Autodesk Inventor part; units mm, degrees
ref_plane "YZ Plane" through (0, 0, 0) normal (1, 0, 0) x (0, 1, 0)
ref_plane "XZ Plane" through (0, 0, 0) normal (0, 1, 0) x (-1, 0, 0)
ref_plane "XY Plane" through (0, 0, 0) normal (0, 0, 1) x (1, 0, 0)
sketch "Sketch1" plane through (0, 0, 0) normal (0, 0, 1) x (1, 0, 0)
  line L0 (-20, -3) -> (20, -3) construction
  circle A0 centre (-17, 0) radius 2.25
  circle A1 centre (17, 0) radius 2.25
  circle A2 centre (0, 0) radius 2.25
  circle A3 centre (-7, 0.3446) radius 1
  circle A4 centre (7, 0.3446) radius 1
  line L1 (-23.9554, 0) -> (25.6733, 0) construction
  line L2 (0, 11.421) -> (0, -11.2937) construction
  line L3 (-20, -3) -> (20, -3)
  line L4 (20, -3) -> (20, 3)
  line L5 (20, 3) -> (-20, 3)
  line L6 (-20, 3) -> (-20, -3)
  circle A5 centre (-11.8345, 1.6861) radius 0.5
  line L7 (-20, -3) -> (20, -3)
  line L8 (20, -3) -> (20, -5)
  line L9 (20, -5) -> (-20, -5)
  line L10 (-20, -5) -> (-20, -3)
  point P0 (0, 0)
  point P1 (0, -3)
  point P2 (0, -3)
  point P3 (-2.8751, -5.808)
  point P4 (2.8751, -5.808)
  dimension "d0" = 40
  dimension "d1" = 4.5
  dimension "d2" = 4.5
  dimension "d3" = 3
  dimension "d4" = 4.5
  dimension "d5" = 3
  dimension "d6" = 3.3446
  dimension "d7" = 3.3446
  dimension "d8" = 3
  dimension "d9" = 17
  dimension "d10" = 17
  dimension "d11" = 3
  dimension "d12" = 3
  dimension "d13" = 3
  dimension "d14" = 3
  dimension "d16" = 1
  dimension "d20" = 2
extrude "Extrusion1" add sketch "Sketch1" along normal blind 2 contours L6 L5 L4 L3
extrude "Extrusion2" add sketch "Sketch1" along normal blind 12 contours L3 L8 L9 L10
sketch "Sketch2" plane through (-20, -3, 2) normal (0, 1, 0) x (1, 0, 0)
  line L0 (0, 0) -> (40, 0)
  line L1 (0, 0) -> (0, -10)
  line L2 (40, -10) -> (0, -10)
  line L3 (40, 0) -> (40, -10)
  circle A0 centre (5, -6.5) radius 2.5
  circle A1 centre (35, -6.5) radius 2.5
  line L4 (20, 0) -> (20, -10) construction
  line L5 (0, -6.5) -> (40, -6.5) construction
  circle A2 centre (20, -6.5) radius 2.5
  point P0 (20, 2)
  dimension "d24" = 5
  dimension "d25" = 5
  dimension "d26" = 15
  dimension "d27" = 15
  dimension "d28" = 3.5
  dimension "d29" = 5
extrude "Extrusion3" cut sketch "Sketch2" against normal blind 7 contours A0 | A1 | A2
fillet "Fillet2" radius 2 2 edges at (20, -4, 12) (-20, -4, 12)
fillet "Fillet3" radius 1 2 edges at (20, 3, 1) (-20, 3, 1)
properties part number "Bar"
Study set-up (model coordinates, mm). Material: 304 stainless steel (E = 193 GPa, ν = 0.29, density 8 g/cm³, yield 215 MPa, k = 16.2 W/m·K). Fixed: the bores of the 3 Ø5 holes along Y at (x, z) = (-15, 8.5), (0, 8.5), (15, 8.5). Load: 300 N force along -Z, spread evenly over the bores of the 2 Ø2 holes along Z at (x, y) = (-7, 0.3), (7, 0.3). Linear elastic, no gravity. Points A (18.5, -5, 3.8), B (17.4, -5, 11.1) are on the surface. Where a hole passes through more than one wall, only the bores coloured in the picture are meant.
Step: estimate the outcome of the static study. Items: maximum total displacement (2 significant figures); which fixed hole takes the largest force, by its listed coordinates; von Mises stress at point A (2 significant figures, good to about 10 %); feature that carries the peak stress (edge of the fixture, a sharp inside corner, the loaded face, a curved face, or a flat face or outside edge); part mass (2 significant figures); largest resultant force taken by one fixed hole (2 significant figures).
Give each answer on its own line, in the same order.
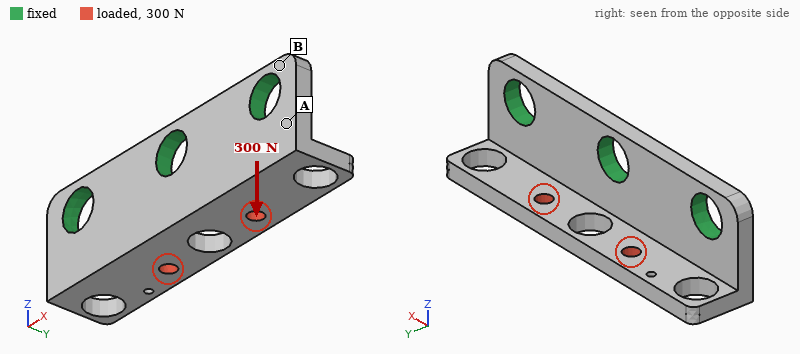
17 µm
(0, 8.5)
34 MPa
the loaded face
9.7 g
180 N
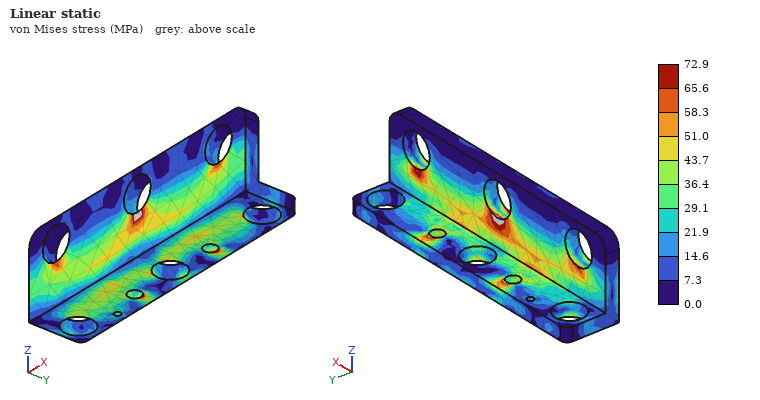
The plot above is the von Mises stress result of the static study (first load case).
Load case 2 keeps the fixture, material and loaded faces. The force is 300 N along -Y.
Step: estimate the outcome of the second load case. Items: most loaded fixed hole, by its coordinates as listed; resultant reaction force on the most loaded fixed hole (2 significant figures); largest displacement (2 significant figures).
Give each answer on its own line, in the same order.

(0, 8.5)
150 N
10 µm
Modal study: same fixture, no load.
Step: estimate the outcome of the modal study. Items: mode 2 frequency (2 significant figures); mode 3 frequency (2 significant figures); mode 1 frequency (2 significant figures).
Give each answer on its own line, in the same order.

17 kHz
29 kHz
14 kHz
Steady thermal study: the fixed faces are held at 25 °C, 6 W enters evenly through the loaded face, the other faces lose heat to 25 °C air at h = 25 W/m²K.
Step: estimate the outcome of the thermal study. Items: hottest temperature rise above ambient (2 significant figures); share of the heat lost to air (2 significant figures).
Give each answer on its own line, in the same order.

77 K
14 %
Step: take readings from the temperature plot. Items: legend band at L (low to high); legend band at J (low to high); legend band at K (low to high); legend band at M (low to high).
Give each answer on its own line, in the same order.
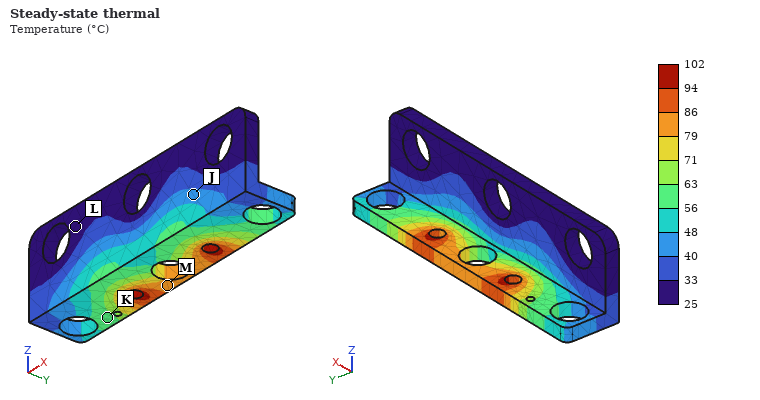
25 to 33 °C
40 to 48 °C
56 to 63 °C
79 to 86 °C
